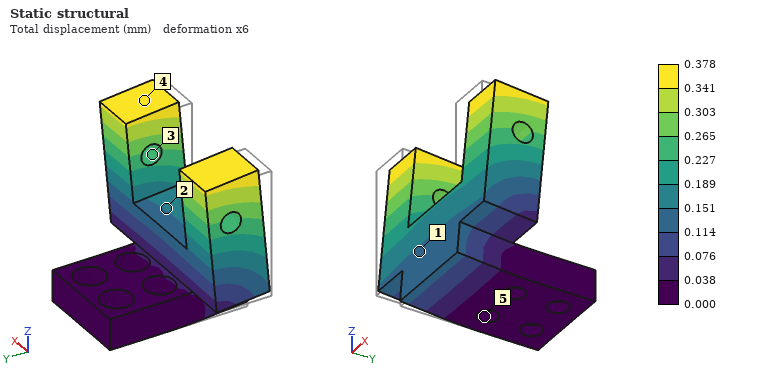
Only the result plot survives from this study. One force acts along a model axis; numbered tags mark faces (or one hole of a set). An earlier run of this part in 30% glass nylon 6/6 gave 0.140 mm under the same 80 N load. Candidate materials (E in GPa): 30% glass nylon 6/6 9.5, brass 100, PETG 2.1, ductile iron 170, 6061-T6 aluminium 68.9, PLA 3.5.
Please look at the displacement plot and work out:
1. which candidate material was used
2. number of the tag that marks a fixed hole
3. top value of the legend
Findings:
PLA
5
0.378 mm
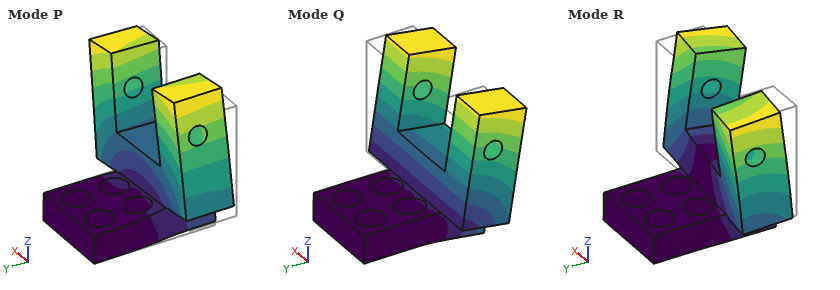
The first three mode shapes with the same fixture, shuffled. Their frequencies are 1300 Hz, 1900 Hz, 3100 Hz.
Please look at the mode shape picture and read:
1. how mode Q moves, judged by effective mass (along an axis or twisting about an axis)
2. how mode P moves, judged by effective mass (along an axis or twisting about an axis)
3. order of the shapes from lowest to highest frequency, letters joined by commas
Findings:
along Y
along X
Q, P, R
